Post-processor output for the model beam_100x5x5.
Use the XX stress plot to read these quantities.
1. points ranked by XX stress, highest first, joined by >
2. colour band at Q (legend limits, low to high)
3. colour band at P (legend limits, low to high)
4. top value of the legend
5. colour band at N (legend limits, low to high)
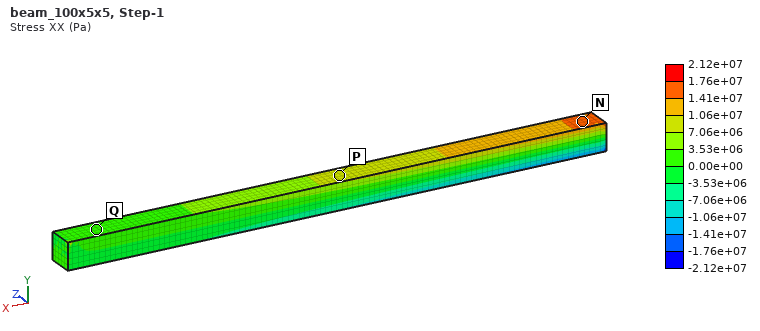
N > P > Q
0.00e+00 to 3.53e+06 Pa
7.06e+06 to 1.06e+07 Pa
2.12e+07 Pa
1.41e+07 to 1.76e+07 Pa
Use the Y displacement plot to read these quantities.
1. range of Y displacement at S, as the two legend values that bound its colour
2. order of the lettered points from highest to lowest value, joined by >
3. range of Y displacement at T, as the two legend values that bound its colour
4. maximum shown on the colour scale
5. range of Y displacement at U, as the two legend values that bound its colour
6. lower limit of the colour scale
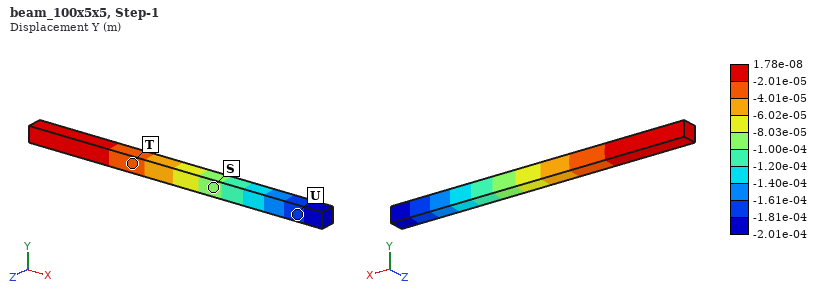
-1.00e-04 to -8.03e-05 m
T > S > U
-4.01e-05 to -2.01e-05 m
1.78e-08 m
-1.81e-04 to -1.61e-04 m
-2.01e-04 m
